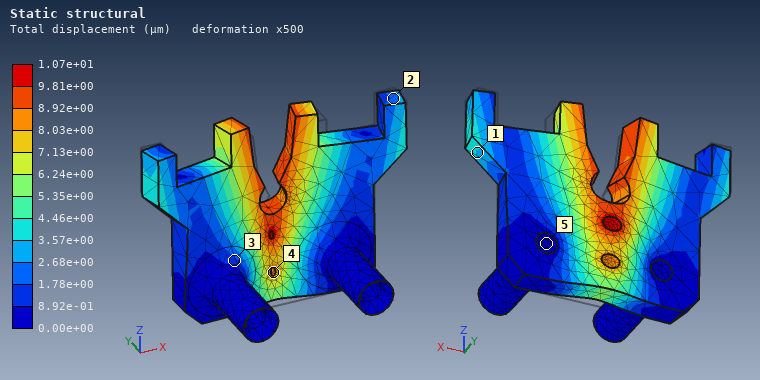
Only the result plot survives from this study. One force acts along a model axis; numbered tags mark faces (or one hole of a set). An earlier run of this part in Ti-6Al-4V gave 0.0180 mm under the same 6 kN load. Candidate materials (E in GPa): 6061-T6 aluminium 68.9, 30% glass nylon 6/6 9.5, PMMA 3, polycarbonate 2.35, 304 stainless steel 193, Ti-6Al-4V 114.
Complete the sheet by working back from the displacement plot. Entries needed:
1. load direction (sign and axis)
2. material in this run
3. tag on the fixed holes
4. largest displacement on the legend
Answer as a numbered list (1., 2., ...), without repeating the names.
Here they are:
1. +Y
2. 304 stainless steel
3. 5
4. 1.07e+01 µm
